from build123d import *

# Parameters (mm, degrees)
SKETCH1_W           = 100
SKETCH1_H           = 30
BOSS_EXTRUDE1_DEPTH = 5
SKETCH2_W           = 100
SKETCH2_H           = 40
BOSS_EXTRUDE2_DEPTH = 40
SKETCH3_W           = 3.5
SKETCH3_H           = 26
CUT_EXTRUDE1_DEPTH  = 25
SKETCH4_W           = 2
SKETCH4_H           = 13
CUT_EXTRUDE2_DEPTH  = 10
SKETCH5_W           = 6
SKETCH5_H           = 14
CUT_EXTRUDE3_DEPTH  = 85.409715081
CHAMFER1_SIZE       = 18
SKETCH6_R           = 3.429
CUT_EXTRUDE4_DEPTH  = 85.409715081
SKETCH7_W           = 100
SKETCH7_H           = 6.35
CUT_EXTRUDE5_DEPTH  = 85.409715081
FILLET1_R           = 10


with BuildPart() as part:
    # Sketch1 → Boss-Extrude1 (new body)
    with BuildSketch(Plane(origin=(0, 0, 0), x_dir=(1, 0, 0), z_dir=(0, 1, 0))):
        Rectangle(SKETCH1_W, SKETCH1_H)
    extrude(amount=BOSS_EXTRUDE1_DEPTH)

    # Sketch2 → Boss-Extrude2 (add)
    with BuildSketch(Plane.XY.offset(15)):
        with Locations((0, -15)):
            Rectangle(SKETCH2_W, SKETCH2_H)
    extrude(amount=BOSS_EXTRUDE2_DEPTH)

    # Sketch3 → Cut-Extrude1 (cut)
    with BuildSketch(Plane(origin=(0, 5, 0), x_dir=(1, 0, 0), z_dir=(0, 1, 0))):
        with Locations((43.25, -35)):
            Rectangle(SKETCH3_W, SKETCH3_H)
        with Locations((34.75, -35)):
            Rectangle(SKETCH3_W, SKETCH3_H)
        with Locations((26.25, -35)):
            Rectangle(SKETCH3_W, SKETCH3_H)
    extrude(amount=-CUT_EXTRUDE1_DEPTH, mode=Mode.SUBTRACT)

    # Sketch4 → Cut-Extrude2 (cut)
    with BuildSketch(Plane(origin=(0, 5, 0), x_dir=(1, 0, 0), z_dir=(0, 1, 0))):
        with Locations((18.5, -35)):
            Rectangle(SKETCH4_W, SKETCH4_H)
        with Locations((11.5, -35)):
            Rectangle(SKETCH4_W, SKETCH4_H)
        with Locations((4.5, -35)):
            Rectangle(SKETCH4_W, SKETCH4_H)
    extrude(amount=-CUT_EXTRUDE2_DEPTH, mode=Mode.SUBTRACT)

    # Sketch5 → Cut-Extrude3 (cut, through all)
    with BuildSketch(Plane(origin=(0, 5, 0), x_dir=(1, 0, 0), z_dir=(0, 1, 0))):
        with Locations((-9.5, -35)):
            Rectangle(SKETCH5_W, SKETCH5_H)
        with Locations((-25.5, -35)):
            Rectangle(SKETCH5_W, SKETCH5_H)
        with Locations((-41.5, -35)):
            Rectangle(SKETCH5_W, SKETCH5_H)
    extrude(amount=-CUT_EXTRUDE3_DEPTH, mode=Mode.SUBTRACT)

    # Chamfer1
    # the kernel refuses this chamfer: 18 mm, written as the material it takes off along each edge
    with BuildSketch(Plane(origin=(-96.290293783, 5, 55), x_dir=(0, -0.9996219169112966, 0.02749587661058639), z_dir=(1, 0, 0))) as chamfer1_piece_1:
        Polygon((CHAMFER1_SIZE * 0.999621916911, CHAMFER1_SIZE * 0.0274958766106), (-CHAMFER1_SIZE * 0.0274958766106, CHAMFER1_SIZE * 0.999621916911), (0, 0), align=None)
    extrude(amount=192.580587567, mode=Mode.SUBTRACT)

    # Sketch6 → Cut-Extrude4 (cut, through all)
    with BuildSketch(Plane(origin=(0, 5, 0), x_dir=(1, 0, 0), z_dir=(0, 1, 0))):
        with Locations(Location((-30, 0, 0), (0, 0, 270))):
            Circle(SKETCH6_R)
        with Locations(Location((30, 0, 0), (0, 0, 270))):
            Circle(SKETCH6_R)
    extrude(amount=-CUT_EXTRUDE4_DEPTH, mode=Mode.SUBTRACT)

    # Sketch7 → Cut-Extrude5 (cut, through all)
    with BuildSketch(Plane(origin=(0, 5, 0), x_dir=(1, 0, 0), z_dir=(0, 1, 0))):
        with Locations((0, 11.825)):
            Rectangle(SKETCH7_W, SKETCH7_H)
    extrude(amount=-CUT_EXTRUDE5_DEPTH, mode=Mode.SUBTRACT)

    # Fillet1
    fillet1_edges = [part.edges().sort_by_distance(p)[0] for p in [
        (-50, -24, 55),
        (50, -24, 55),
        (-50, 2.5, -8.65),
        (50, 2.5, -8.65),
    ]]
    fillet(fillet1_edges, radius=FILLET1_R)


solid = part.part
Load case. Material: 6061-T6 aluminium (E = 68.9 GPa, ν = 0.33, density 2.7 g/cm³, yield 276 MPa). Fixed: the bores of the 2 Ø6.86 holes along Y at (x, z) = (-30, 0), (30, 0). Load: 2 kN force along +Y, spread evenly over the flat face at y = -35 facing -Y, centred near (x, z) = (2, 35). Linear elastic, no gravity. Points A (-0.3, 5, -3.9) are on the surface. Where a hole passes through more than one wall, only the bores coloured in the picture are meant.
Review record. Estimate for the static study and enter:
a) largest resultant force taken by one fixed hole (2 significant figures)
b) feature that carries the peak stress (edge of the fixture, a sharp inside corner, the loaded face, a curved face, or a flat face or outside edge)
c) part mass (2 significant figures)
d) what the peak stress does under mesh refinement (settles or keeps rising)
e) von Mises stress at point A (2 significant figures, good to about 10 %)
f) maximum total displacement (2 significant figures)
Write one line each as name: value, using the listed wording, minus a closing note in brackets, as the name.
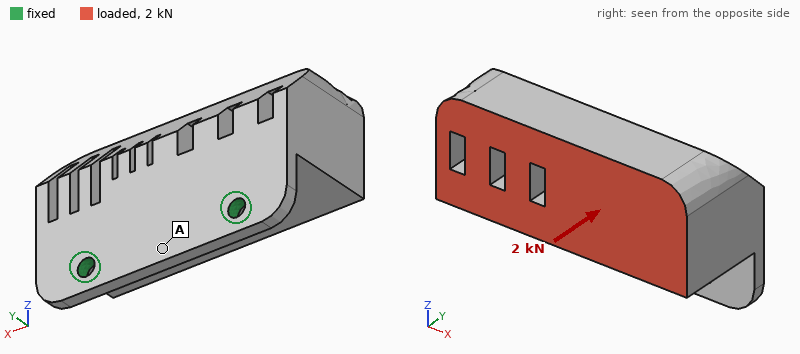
largest resultant force taken by one fixed hole: 1.1 kN
feature that carries the peak stress: edge of the fixture
part mass: 370 g
what the peak stress does under mesh refinement: keeps rising
von Mises stress at point A: 33 MPa
maximum total displacement: 0.88 mm
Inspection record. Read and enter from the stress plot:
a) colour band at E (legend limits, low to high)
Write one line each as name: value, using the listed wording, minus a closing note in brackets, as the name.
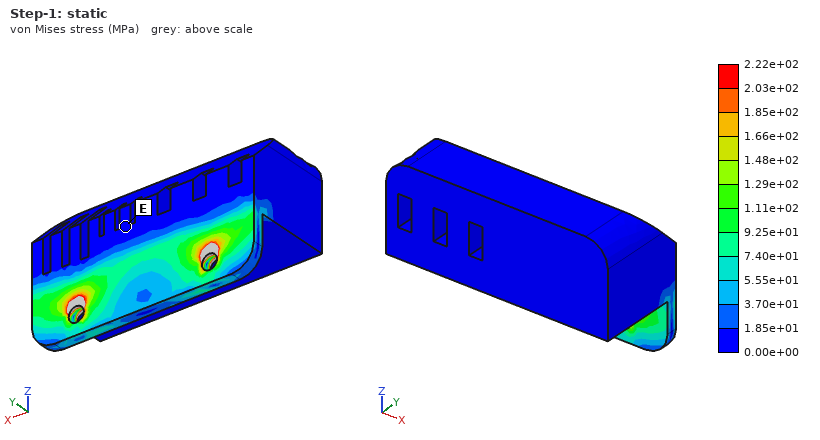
colour band at E: 0.00e+00 to 1.85e+01 MPa
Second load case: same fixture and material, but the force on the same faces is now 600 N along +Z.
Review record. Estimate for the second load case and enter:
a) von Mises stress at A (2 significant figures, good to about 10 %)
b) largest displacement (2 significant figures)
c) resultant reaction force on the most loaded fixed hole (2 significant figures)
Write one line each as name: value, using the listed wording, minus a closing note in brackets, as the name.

von Mises stress at A: 17 MPa
largest displacement: 0.36 mm
resultant reaction force on the most loaded fixed hole: 320 N
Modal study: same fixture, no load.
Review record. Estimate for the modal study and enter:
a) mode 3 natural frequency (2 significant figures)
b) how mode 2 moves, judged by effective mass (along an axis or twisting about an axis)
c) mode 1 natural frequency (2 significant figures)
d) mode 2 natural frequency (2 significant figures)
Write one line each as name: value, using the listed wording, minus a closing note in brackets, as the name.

mode 3 natural frequency: 3600 Hz
how mode 2 moves, judged by effective mass: along X
mode 1 natural frequency: 470 Hz
mode 2 natural frequency: 2100 Hz
